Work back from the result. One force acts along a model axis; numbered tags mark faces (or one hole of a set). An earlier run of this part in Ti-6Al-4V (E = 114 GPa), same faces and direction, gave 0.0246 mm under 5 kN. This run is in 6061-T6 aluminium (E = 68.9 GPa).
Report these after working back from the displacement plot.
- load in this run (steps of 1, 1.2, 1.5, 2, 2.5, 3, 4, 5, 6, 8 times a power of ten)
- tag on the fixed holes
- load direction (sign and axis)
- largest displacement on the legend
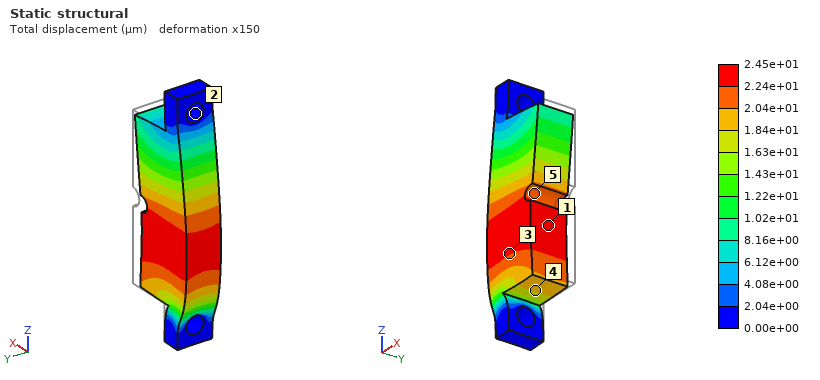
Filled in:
3 kN
2
-X
2.45e+01 µm
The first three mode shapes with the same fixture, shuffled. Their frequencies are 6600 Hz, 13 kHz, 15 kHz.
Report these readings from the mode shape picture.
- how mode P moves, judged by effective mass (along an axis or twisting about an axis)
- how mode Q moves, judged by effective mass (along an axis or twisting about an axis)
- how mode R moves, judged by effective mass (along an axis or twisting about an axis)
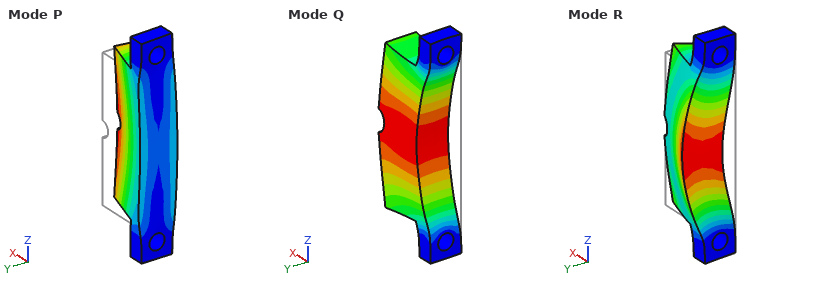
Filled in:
along Y
along X
along Y
